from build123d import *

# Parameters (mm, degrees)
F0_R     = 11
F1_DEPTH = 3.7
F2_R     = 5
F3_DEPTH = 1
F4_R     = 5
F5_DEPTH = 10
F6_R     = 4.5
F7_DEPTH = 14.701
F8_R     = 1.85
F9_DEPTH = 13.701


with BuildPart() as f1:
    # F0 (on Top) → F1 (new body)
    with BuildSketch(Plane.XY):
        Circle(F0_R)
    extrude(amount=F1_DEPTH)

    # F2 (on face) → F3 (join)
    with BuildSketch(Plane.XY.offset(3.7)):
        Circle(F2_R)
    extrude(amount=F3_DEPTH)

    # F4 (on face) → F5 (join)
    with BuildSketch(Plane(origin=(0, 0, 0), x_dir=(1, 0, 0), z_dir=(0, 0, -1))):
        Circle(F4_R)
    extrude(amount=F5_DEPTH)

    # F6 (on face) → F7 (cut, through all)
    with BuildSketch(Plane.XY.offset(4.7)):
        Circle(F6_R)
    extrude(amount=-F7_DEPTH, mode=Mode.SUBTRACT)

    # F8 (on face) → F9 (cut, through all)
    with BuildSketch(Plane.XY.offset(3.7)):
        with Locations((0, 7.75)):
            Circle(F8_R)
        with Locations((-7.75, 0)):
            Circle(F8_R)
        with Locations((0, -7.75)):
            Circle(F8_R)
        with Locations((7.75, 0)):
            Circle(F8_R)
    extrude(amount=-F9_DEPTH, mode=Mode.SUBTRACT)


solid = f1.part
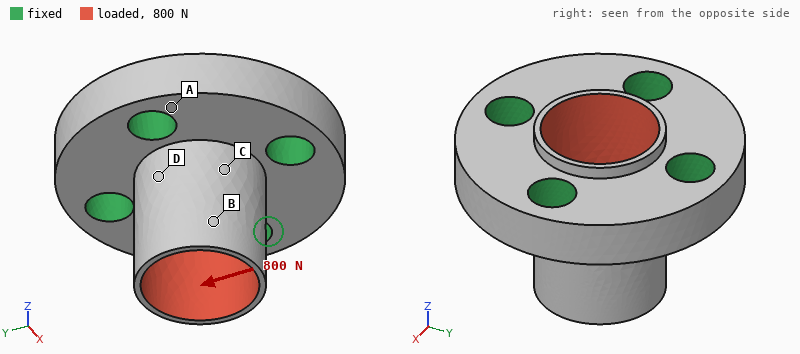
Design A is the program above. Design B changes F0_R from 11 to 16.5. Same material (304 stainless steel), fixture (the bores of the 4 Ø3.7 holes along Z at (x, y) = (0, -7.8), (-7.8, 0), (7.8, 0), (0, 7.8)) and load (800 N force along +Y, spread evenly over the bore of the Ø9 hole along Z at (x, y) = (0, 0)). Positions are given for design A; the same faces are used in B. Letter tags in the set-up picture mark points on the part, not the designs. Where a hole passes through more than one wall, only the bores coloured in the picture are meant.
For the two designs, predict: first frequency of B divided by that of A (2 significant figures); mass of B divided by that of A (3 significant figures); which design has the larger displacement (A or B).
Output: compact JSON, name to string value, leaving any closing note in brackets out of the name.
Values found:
{"first frequency of B divided by that of A": "0.62", "mass of B divided by that of A": "2.49", "which design has the larger displacement": "A"}
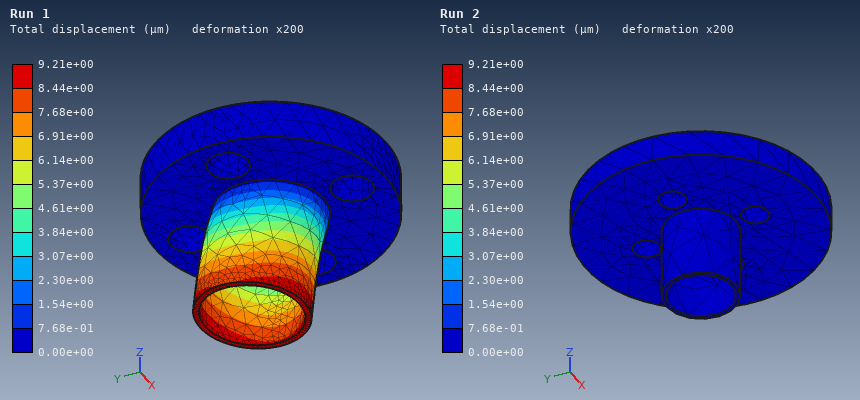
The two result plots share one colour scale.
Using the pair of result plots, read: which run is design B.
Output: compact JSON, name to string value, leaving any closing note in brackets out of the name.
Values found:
{"which run is design B": "Run 2"}
